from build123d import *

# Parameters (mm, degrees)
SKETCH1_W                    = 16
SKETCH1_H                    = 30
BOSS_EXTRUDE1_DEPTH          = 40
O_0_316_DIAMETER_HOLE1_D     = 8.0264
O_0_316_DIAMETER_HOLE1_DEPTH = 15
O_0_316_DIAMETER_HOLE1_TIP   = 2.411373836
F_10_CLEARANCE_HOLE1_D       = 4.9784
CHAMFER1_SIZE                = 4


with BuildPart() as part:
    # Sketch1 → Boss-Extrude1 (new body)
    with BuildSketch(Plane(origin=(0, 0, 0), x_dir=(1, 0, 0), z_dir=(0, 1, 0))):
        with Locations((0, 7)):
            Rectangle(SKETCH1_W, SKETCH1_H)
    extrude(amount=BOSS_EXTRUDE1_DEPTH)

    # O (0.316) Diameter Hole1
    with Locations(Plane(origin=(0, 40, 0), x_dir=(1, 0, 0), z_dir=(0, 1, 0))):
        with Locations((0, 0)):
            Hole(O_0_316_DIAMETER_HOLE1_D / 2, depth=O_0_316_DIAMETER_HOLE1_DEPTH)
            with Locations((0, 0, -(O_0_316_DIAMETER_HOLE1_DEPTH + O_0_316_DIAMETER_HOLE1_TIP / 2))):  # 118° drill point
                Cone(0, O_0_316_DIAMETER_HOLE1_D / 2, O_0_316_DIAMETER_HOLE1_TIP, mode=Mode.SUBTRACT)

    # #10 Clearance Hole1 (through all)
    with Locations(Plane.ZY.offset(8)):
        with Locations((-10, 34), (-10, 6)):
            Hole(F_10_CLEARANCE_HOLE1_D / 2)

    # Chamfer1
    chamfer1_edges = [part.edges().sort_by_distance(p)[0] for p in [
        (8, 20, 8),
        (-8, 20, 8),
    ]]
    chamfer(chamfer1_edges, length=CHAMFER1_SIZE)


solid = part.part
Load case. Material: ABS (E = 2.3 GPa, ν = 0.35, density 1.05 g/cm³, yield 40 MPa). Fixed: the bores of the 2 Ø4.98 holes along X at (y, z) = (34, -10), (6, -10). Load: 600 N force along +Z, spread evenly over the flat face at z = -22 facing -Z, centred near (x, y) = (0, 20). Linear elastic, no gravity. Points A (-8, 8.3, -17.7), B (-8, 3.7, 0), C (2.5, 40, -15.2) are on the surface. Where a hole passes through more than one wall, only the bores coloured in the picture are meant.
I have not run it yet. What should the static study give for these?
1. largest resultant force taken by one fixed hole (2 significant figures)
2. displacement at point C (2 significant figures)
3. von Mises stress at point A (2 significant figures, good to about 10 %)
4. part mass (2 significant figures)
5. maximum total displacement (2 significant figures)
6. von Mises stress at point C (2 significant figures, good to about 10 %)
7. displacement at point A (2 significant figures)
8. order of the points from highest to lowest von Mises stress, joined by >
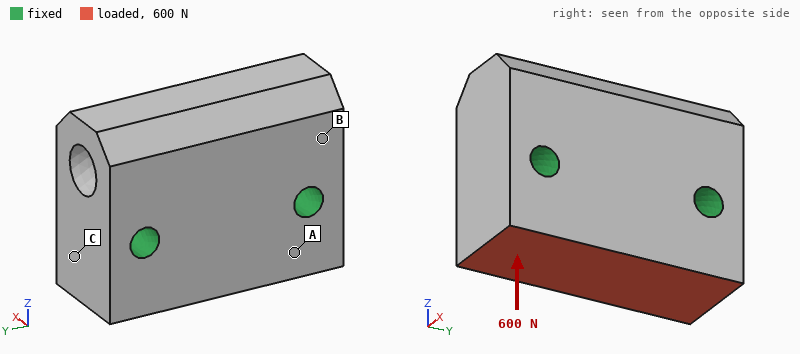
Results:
300 N
2.7 µm
1.1 MPa
18 g
9.1 µm
0.56 MPa
4.1 µm
A > C > B
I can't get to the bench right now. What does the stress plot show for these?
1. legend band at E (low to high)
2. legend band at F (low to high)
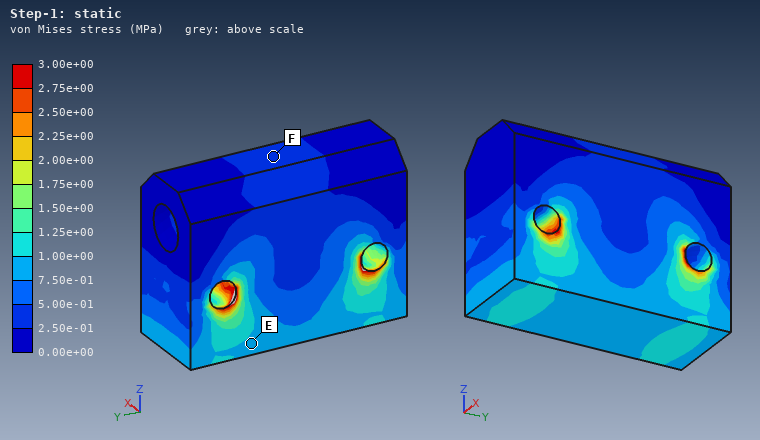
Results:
7.50e-01 to 1.00e+00 MPa
2.50e-01 to 5.00e-01 MPa
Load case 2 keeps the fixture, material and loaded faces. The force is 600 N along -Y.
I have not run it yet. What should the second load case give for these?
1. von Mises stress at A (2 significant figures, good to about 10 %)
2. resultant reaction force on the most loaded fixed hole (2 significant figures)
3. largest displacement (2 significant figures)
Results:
2.0 MPa
370 N
26 µm
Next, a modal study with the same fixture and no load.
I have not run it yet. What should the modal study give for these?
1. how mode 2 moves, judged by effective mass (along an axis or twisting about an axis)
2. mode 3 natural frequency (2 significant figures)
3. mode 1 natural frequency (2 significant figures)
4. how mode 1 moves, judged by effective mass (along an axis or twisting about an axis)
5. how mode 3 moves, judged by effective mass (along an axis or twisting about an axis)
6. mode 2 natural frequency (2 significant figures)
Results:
twisting about Z
11 kHz
7100 Hz
along X
along Y
10 kHz
